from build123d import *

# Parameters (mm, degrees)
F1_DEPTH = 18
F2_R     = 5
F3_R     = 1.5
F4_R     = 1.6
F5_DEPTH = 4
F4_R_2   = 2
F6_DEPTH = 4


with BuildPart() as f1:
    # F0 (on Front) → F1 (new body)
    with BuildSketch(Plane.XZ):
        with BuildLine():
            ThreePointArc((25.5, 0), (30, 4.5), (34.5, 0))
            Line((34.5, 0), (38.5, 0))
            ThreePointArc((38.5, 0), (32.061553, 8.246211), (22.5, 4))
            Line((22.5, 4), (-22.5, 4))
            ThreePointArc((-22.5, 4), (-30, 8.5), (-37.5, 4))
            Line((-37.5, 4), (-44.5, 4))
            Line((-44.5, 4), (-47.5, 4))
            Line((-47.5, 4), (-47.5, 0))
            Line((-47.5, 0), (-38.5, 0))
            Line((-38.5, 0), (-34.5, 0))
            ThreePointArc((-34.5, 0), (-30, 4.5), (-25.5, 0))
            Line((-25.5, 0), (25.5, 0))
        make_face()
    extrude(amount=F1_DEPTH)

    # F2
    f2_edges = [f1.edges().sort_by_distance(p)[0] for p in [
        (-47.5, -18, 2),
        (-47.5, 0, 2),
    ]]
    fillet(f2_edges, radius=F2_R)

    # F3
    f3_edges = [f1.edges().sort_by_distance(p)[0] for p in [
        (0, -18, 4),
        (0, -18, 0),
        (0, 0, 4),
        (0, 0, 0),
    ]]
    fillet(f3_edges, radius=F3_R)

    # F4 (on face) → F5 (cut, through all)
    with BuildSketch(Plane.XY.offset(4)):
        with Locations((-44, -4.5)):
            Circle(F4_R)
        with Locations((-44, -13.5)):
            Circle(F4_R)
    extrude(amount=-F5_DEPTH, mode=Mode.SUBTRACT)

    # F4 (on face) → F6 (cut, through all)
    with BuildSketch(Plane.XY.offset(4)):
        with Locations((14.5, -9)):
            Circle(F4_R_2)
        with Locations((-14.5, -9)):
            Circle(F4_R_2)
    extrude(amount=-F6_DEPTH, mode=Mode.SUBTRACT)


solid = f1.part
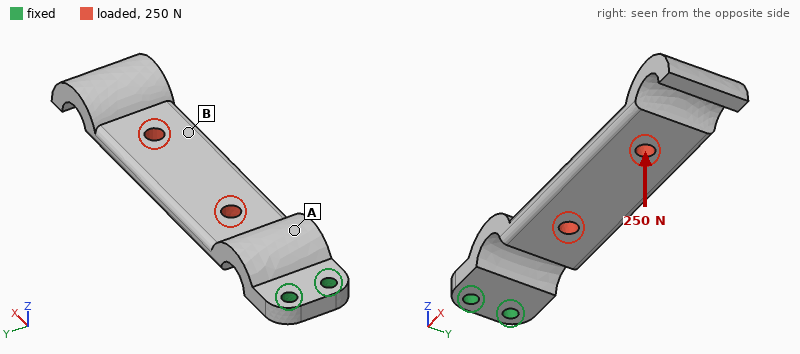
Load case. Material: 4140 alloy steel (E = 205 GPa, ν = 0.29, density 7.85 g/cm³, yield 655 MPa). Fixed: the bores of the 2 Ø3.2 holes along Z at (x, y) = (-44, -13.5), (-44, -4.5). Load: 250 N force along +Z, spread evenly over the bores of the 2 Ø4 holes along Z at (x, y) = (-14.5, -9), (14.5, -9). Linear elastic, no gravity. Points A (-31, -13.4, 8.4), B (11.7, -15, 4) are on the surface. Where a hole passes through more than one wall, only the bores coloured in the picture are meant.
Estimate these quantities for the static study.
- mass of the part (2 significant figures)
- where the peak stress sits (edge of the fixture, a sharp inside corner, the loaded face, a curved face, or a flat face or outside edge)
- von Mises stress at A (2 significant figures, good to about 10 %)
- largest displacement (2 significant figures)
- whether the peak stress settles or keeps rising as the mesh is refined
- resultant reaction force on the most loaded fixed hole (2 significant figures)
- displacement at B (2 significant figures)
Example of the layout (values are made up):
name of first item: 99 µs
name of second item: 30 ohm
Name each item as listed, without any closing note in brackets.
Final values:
mass of the part: 51 g
where the peak stress sits: edge of the fixture
von Mises stress at A: 120 MPa
largest displacement: 0.94 mm
whether the peak stress settles or keeps rising as the mesh is refined: keeps rising
resultant reaction force on the most loaded fixed hole: 130 N
displacement at B: 0.55 mm
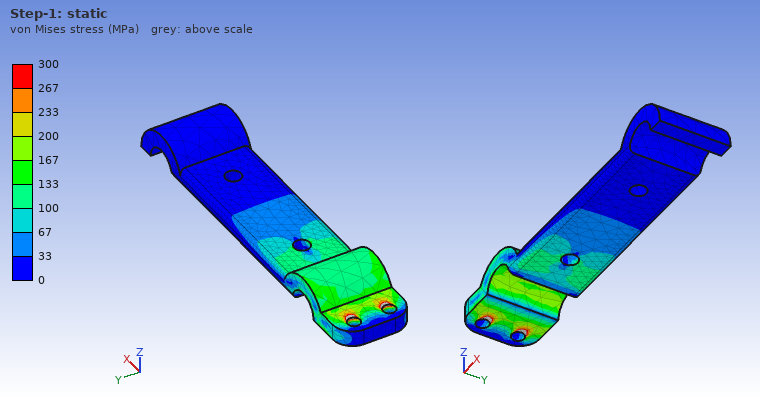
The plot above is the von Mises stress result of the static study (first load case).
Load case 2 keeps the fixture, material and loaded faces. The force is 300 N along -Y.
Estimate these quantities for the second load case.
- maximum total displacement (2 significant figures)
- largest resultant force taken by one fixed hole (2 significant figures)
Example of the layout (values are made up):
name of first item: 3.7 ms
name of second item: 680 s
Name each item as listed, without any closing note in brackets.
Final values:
maximum total displacement: 0.12 mm
largest resultant force taken by one fixed hole: 1.2 kN
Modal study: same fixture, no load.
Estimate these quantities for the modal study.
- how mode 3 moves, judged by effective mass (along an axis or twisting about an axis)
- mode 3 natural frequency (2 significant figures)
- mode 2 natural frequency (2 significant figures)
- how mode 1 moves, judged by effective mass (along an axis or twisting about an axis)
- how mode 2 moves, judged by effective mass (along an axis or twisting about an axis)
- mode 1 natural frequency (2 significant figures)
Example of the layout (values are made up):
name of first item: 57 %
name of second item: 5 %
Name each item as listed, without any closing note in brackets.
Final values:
how mode 3 moves, judged by effective mass: along Z
mode 3 natural frequency: 2800 Hz
mode 2 natural frequency: 1400 Hz
how mode 1 moves, judged by effective mass: along Z
how mode 2 moves, judged by effective mass: along Y
mode 1 natural frequency: 440 Hz
